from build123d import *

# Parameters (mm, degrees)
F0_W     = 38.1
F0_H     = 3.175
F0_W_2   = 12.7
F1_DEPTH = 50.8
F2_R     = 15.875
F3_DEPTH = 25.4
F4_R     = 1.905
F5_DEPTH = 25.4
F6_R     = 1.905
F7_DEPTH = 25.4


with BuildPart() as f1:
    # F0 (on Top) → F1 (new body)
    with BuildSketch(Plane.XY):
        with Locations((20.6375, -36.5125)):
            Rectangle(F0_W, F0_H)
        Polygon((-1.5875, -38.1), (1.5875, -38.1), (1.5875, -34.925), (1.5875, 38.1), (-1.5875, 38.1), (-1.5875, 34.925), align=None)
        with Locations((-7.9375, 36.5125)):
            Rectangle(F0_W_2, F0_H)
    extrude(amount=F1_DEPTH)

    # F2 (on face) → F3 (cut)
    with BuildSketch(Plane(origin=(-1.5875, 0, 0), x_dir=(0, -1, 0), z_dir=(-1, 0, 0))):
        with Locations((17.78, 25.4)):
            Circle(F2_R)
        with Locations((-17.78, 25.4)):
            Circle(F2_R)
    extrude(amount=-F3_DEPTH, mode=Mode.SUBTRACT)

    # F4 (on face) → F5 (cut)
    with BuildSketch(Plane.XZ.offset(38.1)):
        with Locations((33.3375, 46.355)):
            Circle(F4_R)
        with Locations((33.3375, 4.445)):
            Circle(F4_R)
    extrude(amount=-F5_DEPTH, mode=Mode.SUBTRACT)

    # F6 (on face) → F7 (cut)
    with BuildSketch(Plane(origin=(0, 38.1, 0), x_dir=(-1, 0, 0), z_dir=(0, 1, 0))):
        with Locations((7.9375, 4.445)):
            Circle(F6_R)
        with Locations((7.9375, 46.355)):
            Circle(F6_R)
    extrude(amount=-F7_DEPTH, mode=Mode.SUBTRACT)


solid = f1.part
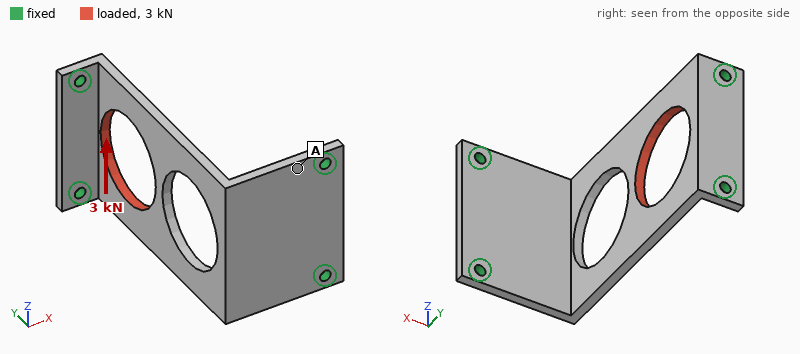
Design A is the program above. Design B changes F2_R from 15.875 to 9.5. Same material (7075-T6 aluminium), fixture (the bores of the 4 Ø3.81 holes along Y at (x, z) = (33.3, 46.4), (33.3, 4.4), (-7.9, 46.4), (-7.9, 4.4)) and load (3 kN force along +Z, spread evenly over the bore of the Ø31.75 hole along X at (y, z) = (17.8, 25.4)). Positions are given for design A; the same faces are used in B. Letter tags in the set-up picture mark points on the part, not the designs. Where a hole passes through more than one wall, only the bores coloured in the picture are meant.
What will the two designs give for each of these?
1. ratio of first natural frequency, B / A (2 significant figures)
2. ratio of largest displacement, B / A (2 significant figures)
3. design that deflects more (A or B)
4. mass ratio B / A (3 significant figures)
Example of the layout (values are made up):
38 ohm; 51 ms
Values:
0.96; 0.42; A; 1.21
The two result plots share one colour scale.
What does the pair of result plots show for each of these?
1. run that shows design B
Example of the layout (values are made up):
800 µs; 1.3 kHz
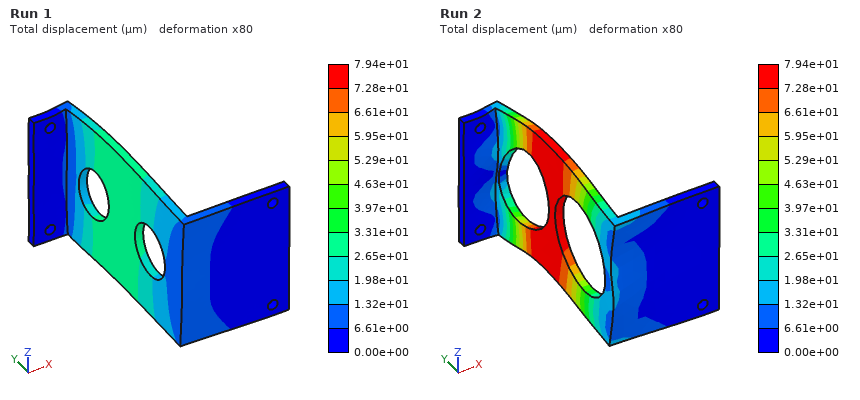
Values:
Run 1
